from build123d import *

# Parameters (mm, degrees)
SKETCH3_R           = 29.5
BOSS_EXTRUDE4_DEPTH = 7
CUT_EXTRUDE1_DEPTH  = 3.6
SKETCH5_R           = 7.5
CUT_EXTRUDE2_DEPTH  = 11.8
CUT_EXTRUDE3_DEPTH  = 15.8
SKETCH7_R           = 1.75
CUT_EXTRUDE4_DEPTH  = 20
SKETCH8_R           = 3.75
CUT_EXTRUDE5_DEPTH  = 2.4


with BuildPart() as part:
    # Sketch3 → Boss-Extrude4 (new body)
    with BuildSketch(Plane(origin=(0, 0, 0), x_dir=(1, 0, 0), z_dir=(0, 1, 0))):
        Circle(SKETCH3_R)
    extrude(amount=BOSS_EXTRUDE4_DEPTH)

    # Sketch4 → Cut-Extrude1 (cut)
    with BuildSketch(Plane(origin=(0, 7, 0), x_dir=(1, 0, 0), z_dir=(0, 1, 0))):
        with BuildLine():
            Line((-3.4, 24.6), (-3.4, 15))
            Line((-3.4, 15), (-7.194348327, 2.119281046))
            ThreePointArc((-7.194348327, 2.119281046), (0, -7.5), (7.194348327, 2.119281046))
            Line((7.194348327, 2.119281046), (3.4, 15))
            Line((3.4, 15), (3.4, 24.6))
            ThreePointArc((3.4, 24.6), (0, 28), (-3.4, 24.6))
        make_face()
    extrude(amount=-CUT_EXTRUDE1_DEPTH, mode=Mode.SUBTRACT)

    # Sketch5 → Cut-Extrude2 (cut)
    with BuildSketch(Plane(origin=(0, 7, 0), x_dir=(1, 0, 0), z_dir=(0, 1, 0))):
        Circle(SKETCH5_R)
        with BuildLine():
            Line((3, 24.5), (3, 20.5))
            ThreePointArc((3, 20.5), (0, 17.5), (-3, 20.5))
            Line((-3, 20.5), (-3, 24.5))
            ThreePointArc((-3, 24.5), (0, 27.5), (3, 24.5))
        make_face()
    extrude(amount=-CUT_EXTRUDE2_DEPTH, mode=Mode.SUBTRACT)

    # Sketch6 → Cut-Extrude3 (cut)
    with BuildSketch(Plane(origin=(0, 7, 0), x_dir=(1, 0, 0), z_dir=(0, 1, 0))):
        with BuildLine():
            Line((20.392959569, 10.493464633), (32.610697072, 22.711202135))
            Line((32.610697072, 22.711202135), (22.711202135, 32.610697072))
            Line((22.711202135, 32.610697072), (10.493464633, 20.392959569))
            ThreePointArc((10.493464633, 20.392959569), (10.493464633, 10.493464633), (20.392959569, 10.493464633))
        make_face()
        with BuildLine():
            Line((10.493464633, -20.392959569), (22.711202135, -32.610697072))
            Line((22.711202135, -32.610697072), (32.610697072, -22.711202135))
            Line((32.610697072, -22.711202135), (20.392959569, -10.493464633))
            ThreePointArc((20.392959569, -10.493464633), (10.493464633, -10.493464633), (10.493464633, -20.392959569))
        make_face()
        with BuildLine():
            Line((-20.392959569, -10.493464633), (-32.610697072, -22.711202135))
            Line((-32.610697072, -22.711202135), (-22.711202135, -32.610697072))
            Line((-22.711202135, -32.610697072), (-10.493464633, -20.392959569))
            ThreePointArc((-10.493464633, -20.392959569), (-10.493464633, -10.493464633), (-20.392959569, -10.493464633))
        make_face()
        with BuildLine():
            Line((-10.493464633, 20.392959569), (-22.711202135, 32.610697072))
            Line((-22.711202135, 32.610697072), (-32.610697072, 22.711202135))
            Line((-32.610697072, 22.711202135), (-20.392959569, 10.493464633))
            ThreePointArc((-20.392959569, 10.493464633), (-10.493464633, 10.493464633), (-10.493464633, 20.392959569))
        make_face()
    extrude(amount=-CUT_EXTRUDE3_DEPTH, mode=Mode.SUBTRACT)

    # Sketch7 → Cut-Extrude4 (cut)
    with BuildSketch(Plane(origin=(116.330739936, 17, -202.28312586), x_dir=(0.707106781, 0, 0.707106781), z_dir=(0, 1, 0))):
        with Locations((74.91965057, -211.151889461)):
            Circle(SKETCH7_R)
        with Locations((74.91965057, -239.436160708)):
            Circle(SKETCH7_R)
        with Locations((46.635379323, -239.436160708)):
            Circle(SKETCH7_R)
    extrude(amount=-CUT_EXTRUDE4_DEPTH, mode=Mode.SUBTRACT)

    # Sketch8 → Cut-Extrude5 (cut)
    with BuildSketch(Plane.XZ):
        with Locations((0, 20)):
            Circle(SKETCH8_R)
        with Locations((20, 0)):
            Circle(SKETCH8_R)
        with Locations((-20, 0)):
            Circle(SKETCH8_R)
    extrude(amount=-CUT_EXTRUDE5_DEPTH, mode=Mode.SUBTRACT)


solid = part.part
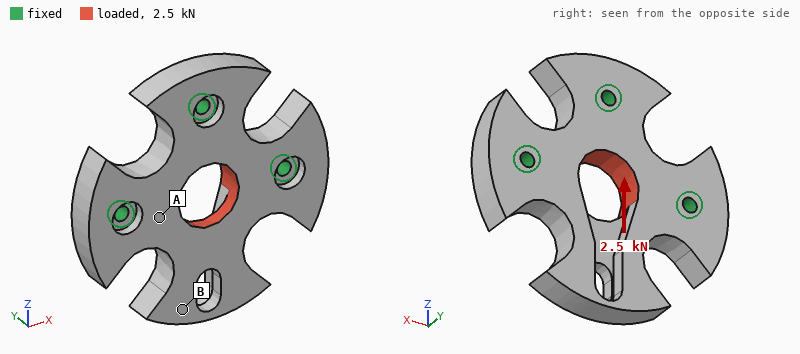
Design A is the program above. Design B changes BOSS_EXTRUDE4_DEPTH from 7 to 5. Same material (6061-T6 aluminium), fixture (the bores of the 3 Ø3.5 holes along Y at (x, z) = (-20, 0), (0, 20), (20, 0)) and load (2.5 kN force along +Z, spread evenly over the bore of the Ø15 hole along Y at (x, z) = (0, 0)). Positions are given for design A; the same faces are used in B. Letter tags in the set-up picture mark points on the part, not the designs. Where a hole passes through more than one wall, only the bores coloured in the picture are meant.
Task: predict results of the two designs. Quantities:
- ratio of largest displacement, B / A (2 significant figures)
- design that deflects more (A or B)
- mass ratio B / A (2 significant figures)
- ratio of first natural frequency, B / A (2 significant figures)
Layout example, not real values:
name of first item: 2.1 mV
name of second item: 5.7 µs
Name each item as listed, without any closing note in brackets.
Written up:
ratio of largest displacement, B / A: 1.8
design that deflects more: B
mass ratio B / A: 0.72
ratio of first natural frequency, B / A: 0.73
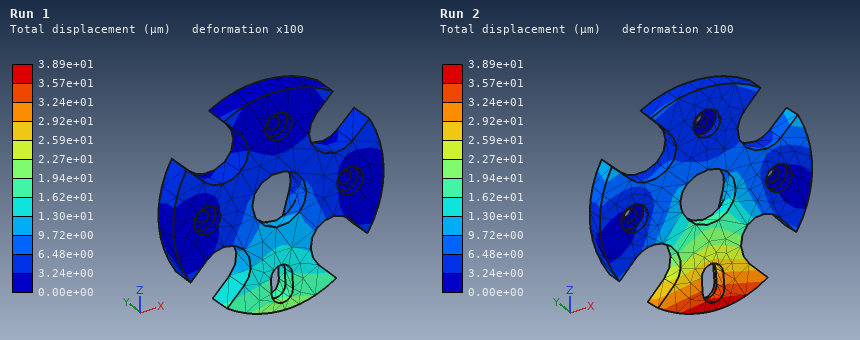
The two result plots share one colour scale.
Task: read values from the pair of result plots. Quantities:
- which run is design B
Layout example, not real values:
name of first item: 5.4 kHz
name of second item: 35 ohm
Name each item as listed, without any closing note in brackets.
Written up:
which run is design B: Run 2
